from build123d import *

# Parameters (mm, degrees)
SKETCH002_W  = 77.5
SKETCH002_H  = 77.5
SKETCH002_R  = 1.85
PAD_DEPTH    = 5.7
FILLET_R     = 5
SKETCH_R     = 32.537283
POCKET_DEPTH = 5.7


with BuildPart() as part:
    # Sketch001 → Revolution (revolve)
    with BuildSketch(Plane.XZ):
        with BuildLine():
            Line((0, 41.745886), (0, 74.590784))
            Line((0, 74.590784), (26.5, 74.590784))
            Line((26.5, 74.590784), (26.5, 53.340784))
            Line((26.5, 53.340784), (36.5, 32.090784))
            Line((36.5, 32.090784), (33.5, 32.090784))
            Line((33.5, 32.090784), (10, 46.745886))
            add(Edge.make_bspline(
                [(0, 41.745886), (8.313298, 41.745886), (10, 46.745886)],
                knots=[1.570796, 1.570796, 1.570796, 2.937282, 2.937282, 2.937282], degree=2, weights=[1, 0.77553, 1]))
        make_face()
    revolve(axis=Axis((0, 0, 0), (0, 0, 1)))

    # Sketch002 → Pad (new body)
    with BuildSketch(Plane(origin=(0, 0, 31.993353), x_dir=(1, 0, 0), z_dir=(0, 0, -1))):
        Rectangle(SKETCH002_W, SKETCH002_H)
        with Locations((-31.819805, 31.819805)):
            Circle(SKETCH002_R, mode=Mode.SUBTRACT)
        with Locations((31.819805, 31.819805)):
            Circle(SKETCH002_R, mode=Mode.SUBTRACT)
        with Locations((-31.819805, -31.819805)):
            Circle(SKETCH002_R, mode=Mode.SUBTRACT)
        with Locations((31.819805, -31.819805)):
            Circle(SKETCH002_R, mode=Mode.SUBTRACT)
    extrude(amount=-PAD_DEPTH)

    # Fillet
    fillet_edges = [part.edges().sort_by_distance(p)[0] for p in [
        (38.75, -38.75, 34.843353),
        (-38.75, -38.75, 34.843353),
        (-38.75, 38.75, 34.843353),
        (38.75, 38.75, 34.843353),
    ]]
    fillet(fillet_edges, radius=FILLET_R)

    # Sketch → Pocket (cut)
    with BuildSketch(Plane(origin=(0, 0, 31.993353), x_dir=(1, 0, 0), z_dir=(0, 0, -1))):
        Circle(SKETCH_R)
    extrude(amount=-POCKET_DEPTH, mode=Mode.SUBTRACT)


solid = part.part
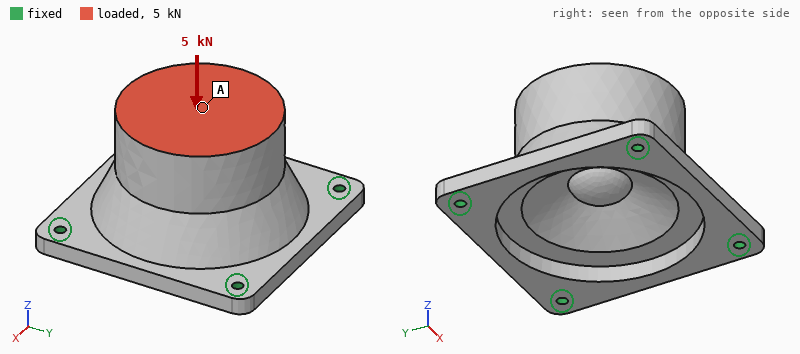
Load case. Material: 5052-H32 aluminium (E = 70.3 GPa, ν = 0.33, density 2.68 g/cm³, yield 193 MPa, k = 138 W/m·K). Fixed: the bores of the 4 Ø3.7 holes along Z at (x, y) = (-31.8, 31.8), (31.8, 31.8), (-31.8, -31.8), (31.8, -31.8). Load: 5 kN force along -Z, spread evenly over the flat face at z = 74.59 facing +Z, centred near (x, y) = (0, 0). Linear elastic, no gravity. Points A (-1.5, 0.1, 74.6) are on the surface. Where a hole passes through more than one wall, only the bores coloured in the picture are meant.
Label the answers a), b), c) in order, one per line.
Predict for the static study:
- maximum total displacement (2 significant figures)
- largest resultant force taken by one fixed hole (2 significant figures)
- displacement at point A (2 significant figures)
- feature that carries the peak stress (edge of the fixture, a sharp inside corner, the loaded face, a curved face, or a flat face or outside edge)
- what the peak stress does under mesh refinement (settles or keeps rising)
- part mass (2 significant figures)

a) 32 µm
b) 1.8 kN
c) 31 µm
d) edge of the fixture
e) keeps rising
f) 260 g
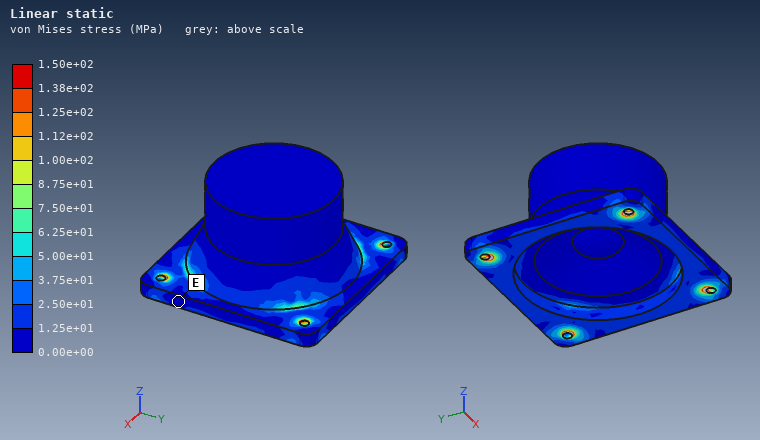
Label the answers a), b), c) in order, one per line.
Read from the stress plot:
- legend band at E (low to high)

a) 0.00e+00 to 1.25e+01 MPa
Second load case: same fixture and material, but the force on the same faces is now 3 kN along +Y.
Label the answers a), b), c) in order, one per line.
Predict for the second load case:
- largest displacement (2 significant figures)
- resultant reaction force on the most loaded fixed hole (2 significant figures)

a) 51 µm
b) 1.6 kN
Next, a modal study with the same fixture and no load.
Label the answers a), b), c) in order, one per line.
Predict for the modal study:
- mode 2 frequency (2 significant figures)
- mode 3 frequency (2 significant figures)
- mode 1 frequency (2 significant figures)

a) 4000 Hz
b) 4100 Hz
c) 4000 Hz
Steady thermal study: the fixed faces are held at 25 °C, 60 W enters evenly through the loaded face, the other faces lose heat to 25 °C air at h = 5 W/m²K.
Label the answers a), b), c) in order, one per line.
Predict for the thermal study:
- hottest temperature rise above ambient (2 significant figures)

a) 26 K
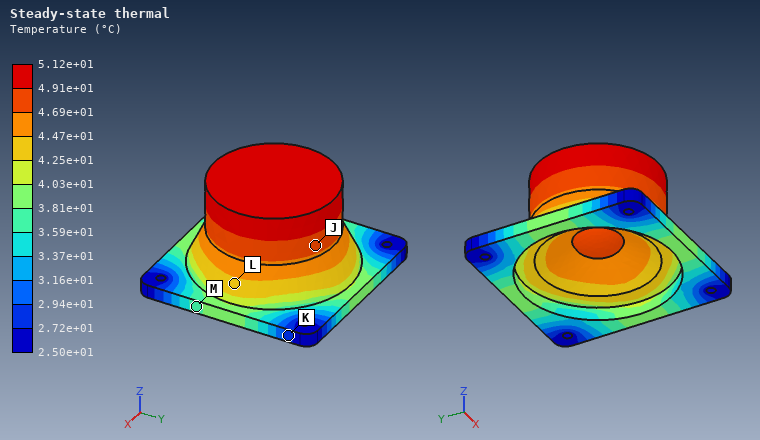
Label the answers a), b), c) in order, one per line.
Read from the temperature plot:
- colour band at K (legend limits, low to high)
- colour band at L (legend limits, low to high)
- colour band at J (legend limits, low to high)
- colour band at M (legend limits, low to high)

a) 2.72e+01 to 2.94e+01 °C
b) 4.25e+01 to 4.47e+01 °C
c) 4.69e+01 to 4.91e+01 °C
d) 3.59e+01 to 3.81e+01 °C
